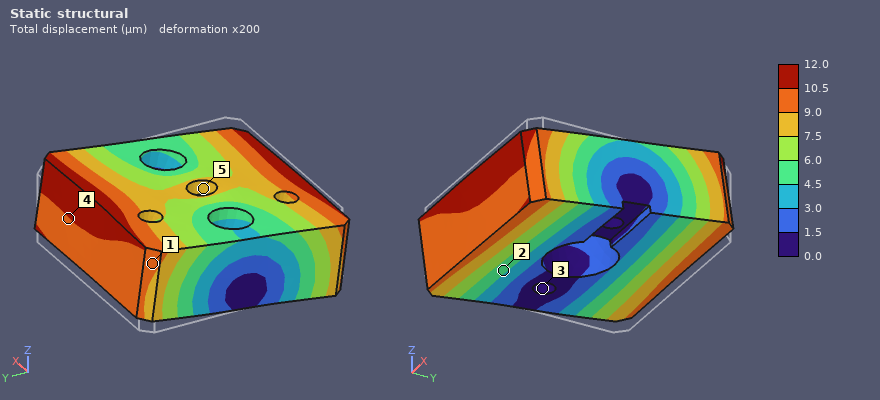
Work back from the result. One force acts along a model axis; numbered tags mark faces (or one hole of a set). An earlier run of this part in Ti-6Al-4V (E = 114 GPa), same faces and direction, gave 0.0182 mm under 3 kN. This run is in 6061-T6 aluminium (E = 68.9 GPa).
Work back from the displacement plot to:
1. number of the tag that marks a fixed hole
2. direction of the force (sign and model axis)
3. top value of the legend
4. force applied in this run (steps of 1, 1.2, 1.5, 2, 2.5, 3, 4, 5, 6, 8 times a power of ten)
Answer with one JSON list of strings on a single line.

["3", "-Y", "12.0 µm", "1.2 kN"]
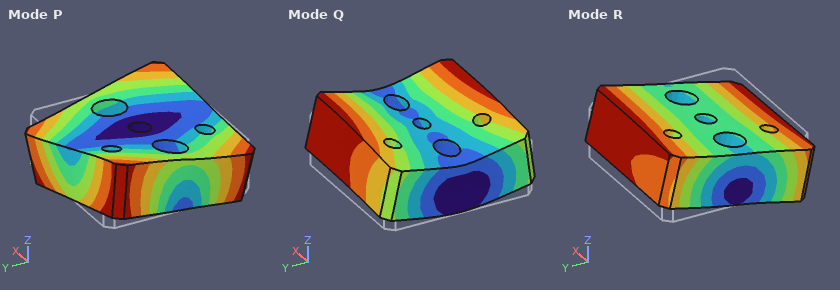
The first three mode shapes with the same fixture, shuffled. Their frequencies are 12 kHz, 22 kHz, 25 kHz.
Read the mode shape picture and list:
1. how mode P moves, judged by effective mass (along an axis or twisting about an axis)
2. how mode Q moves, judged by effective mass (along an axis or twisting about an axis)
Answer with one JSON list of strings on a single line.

["twisting about Z", "along Z"]
